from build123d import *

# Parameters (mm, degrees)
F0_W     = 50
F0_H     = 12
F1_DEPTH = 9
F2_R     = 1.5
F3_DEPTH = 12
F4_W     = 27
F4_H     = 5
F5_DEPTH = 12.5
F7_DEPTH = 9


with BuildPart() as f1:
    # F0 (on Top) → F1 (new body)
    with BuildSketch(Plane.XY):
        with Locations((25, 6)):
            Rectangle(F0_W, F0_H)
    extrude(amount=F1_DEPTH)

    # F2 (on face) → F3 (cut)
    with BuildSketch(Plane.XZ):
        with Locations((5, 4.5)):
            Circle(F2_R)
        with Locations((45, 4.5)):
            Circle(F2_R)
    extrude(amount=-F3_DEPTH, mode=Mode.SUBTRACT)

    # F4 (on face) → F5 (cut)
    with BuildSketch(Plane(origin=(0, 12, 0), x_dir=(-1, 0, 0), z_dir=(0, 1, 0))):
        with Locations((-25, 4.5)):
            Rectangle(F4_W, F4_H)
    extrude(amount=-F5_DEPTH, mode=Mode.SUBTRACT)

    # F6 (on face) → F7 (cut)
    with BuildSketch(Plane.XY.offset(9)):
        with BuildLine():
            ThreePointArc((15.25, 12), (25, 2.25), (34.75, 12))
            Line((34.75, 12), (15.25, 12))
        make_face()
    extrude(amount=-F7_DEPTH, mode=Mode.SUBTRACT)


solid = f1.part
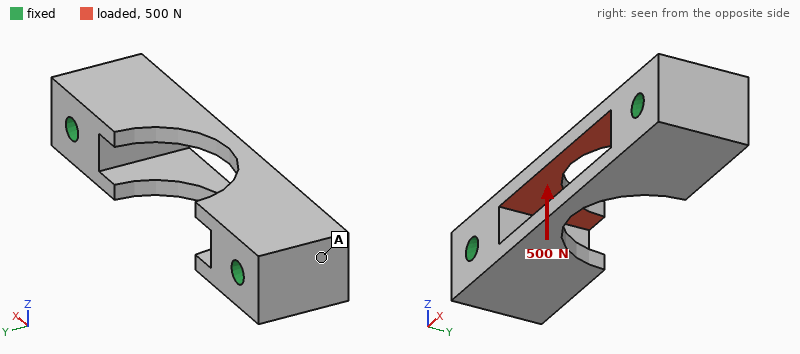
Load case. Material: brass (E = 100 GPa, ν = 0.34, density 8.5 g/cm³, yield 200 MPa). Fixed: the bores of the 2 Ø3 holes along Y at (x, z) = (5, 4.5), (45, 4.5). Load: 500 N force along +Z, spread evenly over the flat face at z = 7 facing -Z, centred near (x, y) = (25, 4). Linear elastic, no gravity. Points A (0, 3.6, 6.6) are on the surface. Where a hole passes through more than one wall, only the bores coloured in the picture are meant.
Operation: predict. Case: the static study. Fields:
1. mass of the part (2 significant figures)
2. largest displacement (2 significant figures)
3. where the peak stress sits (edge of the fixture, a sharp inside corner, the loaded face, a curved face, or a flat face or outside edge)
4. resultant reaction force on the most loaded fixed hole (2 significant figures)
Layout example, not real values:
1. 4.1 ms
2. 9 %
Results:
1. 26 g
2. 64 µm
3. a curved face
4. 250 N
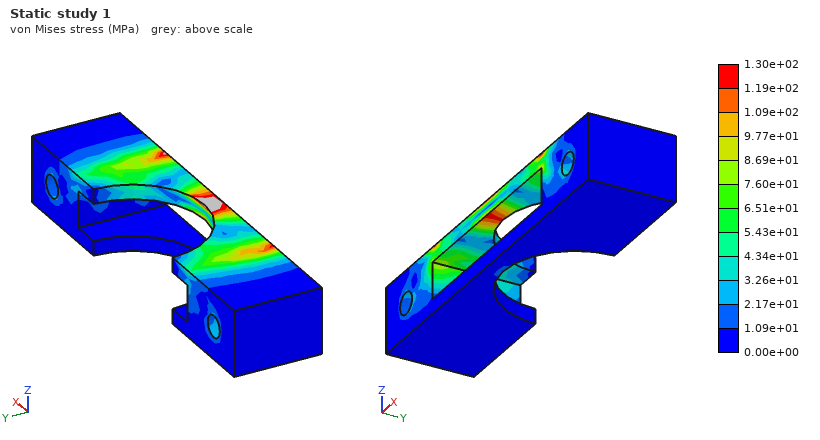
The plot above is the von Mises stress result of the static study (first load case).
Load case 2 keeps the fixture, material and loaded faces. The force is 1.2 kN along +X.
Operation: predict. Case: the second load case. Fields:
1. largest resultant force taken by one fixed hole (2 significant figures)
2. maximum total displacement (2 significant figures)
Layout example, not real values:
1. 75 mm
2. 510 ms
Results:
1. 600 N
2. 5.0 µm
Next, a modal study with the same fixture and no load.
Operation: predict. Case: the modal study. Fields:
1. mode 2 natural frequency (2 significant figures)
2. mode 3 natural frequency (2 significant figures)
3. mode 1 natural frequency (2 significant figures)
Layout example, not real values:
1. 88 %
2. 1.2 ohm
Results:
1. 11 kHz
2. 20 kHz
3. 10 kHz
